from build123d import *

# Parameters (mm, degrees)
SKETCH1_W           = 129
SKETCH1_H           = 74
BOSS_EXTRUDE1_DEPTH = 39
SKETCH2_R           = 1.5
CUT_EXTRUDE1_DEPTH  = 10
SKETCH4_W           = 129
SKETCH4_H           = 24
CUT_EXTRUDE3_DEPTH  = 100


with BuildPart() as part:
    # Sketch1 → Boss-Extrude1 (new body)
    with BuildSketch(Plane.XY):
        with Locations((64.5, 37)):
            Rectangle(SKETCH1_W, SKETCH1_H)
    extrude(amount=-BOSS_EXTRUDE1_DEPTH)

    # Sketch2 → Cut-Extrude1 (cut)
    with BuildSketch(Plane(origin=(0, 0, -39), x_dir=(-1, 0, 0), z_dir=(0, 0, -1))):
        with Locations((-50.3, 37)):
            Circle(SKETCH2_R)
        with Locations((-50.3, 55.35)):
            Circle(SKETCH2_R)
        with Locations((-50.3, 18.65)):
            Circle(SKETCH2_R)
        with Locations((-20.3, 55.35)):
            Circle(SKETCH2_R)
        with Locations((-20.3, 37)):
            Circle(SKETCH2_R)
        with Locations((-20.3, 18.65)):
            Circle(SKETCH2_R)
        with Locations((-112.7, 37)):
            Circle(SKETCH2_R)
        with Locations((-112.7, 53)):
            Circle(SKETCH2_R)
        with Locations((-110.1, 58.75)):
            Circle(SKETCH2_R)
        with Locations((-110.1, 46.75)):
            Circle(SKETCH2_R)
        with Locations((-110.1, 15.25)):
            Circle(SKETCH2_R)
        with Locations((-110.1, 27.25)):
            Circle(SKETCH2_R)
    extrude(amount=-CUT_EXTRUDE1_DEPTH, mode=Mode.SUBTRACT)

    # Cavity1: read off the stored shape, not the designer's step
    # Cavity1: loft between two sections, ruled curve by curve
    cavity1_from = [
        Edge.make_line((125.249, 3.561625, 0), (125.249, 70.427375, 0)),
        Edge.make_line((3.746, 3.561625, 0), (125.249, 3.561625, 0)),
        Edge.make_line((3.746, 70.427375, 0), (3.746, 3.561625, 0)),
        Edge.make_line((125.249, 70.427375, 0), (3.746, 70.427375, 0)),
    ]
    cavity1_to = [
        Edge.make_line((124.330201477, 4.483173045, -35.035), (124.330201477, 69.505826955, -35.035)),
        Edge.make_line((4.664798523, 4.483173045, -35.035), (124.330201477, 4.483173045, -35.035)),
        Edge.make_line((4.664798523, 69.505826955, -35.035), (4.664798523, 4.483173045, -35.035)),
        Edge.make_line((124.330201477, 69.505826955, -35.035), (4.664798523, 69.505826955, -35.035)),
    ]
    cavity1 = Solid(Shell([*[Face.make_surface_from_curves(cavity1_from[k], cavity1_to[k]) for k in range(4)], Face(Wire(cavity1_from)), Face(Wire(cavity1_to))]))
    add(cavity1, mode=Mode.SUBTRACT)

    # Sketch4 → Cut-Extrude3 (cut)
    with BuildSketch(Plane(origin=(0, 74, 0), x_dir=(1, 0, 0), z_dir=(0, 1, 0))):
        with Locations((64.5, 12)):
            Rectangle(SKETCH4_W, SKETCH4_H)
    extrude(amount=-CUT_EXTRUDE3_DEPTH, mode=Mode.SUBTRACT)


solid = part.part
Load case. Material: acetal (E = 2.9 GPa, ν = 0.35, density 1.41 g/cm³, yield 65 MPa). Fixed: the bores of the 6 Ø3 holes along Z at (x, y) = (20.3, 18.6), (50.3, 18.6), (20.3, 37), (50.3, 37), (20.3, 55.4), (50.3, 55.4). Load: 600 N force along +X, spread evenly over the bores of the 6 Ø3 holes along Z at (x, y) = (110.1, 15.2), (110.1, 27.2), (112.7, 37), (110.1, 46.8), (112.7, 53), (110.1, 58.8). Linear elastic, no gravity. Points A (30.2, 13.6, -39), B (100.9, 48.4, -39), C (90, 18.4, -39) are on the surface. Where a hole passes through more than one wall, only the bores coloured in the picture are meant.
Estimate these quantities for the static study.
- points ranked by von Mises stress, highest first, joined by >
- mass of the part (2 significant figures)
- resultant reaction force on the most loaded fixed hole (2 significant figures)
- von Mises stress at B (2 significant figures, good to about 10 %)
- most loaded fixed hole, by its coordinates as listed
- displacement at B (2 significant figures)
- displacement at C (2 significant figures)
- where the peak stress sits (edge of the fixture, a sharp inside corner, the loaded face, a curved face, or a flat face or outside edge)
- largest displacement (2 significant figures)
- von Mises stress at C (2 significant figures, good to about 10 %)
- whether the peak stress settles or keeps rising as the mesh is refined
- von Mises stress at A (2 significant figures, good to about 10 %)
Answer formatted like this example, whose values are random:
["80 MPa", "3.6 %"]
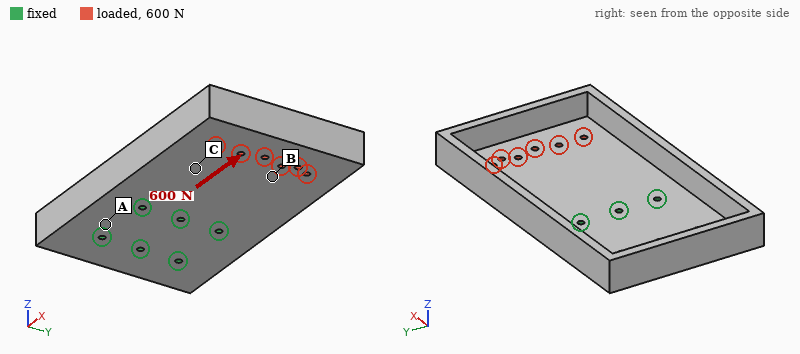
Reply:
["B > C > A", "80 g", "200 N", "3.1 MPa", "(50.3, 55.4)", "0.086 mm", "0.054 mm", "edge of the fixture", "0.17 mm", "2.1 MPa", "keeps rising", "0.58 MPa"]
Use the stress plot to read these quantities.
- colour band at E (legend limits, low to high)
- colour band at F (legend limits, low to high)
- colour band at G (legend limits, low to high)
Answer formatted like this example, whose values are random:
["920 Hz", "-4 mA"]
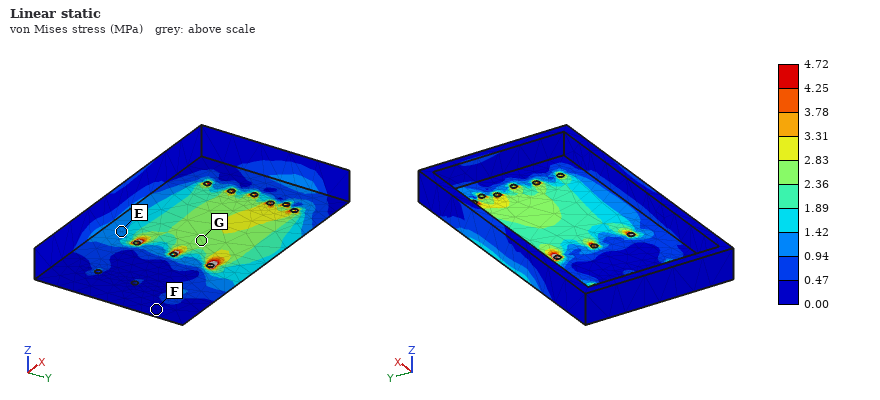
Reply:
["0.94 to 1.42 MPa", "0.00 to 0.47 MPa", "2.36 to 2.83 MPa"]
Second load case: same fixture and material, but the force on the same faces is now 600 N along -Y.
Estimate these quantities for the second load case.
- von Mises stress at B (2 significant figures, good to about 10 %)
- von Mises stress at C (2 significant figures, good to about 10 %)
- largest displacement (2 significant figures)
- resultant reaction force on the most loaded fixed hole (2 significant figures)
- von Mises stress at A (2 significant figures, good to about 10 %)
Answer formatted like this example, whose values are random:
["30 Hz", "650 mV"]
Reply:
["3.5 MPa", "3.2 MPa", "0.61 mm", "590 N", "3.3 MPa"]
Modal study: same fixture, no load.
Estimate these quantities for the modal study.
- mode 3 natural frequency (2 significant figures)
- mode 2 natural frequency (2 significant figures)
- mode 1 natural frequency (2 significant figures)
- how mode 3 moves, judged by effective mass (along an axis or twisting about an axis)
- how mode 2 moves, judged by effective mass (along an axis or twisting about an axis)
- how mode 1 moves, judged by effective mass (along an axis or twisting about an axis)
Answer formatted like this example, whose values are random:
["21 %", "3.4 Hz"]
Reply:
["1200 Hz", "360 Hz", "240 Hz", "along Y", "twisting about X", "along Z"]
